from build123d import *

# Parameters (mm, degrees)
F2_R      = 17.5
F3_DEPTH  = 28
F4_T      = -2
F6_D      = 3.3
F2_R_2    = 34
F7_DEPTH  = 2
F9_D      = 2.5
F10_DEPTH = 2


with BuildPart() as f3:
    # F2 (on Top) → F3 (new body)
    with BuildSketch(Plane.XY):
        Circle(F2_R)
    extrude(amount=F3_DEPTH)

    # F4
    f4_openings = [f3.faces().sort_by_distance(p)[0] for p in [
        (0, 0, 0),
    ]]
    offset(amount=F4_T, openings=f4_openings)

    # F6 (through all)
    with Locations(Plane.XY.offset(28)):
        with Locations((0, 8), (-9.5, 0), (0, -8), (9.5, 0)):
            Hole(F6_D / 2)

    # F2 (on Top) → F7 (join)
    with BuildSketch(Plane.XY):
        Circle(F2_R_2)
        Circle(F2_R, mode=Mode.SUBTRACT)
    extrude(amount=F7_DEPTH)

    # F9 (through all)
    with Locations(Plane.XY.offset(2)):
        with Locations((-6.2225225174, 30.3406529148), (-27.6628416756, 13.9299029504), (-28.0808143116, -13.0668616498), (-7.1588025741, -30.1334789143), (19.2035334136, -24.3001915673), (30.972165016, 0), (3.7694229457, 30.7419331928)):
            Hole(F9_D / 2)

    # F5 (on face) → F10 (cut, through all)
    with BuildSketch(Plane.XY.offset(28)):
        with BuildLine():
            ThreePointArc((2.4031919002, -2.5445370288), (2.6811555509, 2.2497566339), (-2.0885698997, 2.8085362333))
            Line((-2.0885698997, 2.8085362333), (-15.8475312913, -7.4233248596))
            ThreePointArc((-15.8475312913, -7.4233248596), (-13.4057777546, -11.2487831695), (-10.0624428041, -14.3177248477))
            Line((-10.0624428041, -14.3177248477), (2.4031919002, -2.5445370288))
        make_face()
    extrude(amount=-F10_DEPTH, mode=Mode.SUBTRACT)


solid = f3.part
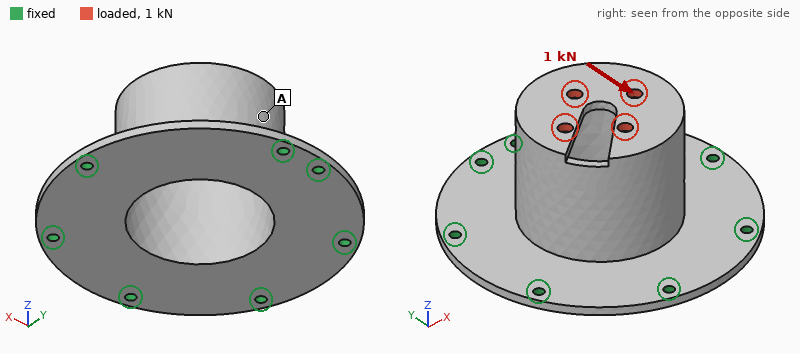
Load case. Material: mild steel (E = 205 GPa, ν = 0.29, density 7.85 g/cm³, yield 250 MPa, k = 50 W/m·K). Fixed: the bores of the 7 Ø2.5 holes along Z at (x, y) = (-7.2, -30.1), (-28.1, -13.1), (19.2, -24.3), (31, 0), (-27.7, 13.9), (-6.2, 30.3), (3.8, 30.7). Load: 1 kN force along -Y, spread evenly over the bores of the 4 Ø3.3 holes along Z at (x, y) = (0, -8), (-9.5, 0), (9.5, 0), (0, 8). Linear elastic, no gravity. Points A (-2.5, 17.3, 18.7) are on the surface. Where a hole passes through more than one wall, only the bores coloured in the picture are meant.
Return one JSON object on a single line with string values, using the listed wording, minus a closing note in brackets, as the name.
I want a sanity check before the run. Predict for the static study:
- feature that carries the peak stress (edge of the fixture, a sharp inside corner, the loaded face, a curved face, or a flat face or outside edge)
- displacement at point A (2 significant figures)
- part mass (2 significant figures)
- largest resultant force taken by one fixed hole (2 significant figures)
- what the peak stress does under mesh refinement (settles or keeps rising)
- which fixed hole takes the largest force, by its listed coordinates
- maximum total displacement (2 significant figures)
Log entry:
{"feature that carries the peak stress": "edge of the fixture", "displacement at point A": "48 µm", "part mass": "96 g", "largest resultant force taken by one fixed hole": "390 N", "what the peak stress does under mesh refinement": "keeps rising", "which fixed hole takes the largest force, by its listed coordinates": "(-7.2, -30.1)", "maximum total displacement": "64 µm"}
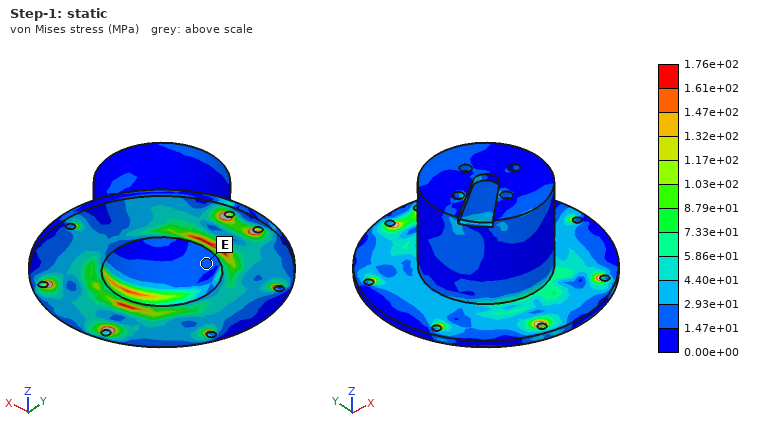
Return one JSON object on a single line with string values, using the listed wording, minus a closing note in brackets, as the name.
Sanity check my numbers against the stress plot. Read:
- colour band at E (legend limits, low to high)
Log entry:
{"colour band at E": "1.47e+01 to 2.93e+01 MPa"}
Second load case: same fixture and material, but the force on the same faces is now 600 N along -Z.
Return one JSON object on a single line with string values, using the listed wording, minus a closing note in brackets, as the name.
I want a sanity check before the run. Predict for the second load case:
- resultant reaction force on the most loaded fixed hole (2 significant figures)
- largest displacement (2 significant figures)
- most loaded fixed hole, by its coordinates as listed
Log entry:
{"resultant reaction force on the most loaded fixed hole": "140 N", "largest displacement": "33 µm", "most loaded fixed hole, by its coordinates as listed": "(31, 0)"}
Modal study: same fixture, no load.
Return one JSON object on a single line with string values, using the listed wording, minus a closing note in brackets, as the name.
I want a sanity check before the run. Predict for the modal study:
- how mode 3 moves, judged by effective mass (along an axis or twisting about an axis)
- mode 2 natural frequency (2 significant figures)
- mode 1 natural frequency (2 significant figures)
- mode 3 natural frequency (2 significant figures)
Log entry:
{"how mode 3 moves, judged by effective mass": "along Z", "mode 2 natural frequency": "3800 Hz", "mode 1 natural frequency": "3500 Hz", "mode 3 natural frequency": "4200 Hz"}
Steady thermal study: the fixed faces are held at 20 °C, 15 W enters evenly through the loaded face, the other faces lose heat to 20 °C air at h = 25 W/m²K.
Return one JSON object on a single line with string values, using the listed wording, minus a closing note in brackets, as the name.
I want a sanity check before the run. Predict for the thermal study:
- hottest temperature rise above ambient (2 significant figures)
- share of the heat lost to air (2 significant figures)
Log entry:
{"hottest temperature rise above ambient": "68 K", "share of the heat lost to air": "41 %"}
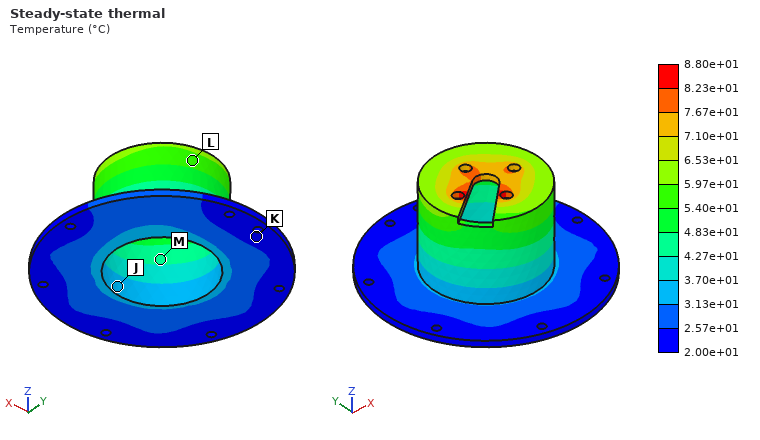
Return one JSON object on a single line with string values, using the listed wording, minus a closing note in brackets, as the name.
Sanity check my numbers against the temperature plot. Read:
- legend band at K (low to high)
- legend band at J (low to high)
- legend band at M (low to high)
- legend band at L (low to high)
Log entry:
{"legend band at K": "2.00e+01 to 2.57e+01 °C", "legend band at J": "3.13e+01 to 3.70e+01 °C", "legend band at M": "4.27e+01 to 4.83e+01 °C", "legend band at L": "5.40e+01 to 5.97e+01 °C"}
